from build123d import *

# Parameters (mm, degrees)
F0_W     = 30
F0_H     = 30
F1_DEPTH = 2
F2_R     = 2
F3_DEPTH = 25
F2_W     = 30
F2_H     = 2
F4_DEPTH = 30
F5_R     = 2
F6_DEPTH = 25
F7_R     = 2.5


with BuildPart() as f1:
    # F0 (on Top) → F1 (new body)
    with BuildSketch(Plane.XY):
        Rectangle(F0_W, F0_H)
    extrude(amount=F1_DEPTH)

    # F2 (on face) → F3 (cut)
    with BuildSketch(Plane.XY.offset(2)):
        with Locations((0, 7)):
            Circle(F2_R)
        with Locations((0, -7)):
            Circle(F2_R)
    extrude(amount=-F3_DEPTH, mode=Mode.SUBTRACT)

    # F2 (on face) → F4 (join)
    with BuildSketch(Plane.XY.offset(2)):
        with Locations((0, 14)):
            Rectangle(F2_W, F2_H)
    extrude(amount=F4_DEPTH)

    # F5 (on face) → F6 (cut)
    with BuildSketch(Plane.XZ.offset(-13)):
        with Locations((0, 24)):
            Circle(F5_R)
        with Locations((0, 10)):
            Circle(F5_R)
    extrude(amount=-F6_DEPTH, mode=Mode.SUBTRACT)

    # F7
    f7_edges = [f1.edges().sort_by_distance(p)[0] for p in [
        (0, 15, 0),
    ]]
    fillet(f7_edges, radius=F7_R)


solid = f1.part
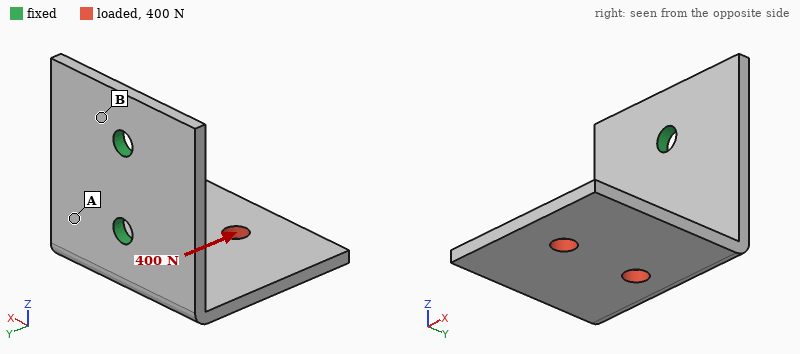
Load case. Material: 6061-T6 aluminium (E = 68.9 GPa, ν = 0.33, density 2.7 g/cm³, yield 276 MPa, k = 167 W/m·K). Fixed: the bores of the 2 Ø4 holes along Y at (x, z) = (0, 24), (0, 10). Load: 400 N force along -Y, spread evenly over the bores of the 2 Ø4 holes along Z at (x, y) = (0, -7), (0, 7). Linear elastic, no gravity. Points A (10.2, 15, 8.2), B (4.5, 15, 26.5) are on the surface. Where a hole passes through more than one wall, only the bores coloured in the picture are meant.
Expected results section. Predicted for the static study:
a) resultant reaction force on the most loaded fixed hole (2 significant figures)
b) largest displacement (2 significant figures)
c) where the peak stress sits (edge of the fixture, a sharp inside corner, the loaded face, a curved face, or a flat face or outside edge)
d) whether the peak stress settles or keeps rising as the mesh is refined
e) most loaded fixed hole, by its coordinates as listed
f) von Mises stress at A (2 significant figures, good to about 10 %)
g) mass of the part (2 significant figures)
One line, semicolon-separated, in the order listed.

470 N; 0.36 mm; edge of the fixture; keeps rising; (0, 10); 61 MPa; 9.3 g
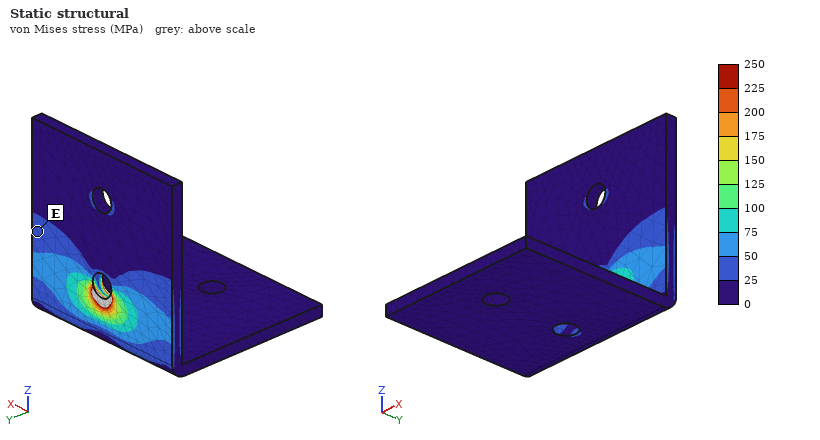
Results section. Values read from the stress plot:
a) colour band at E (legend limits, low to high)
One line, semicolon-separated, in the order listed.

25 to 50 MPa
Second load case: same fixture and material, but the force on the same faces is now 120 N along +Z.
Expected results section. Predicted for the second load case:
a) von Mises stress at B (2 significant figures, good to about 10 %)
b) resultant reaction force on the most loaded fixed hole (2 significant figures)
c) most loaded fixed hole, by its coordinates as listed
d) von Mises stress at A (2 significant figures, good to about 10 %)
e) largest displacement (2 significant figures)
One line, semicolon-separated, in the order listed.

11 MPa; 110 N; (0, 10); 52 MPa; 0.56 mm
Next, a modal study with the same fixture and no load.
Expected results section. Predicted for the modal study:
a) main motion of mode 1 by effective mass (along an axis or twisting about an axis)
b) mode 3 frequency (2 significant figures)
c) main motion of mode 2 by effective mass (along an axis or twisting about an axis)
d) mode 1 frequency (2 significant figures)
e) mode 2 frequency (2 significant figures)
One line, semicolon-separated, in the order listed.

along Z; 4100 Hz; along X; 1300 Hz; 2000 Hz
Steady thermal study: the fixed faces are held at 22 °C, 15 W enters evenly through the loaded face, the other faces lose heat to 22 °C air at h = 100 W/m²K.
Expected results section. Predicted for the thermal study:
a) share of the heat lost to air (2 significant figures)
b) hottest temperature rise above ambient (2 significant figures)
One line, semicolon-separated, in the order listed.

32 %; 32 K
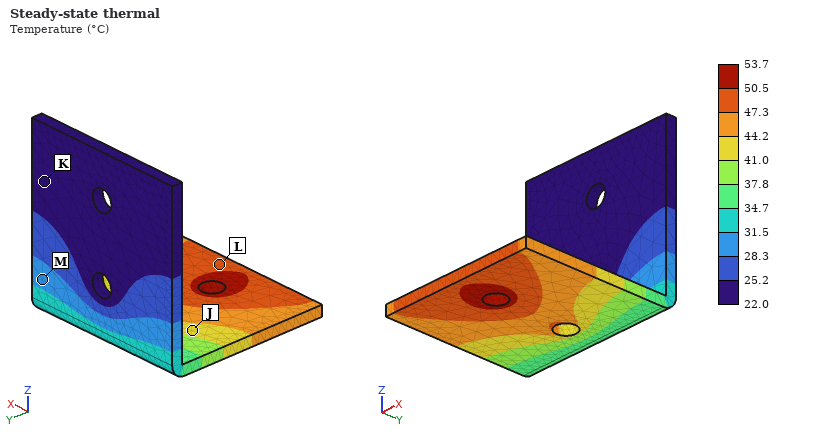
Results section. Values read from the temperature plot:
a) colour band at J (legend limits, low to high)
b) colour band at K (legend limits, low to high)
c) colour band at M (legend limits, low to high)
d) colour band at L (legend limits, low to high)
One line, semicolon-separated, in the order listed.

41.0 to 44.2 °C; 22.0 to 25.2 °C; 28.3 to 31.5 °C; 47.3 to 50.5 °C
